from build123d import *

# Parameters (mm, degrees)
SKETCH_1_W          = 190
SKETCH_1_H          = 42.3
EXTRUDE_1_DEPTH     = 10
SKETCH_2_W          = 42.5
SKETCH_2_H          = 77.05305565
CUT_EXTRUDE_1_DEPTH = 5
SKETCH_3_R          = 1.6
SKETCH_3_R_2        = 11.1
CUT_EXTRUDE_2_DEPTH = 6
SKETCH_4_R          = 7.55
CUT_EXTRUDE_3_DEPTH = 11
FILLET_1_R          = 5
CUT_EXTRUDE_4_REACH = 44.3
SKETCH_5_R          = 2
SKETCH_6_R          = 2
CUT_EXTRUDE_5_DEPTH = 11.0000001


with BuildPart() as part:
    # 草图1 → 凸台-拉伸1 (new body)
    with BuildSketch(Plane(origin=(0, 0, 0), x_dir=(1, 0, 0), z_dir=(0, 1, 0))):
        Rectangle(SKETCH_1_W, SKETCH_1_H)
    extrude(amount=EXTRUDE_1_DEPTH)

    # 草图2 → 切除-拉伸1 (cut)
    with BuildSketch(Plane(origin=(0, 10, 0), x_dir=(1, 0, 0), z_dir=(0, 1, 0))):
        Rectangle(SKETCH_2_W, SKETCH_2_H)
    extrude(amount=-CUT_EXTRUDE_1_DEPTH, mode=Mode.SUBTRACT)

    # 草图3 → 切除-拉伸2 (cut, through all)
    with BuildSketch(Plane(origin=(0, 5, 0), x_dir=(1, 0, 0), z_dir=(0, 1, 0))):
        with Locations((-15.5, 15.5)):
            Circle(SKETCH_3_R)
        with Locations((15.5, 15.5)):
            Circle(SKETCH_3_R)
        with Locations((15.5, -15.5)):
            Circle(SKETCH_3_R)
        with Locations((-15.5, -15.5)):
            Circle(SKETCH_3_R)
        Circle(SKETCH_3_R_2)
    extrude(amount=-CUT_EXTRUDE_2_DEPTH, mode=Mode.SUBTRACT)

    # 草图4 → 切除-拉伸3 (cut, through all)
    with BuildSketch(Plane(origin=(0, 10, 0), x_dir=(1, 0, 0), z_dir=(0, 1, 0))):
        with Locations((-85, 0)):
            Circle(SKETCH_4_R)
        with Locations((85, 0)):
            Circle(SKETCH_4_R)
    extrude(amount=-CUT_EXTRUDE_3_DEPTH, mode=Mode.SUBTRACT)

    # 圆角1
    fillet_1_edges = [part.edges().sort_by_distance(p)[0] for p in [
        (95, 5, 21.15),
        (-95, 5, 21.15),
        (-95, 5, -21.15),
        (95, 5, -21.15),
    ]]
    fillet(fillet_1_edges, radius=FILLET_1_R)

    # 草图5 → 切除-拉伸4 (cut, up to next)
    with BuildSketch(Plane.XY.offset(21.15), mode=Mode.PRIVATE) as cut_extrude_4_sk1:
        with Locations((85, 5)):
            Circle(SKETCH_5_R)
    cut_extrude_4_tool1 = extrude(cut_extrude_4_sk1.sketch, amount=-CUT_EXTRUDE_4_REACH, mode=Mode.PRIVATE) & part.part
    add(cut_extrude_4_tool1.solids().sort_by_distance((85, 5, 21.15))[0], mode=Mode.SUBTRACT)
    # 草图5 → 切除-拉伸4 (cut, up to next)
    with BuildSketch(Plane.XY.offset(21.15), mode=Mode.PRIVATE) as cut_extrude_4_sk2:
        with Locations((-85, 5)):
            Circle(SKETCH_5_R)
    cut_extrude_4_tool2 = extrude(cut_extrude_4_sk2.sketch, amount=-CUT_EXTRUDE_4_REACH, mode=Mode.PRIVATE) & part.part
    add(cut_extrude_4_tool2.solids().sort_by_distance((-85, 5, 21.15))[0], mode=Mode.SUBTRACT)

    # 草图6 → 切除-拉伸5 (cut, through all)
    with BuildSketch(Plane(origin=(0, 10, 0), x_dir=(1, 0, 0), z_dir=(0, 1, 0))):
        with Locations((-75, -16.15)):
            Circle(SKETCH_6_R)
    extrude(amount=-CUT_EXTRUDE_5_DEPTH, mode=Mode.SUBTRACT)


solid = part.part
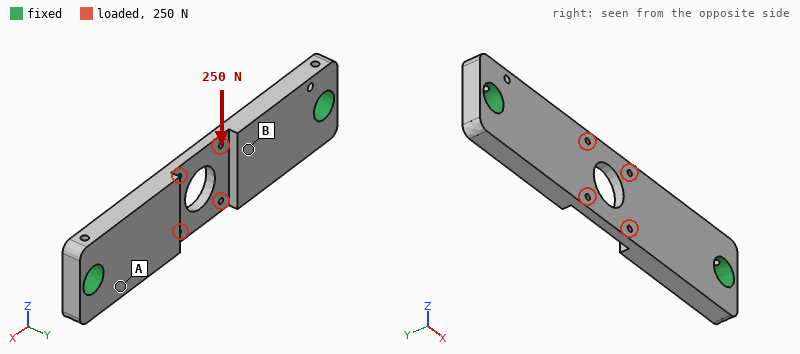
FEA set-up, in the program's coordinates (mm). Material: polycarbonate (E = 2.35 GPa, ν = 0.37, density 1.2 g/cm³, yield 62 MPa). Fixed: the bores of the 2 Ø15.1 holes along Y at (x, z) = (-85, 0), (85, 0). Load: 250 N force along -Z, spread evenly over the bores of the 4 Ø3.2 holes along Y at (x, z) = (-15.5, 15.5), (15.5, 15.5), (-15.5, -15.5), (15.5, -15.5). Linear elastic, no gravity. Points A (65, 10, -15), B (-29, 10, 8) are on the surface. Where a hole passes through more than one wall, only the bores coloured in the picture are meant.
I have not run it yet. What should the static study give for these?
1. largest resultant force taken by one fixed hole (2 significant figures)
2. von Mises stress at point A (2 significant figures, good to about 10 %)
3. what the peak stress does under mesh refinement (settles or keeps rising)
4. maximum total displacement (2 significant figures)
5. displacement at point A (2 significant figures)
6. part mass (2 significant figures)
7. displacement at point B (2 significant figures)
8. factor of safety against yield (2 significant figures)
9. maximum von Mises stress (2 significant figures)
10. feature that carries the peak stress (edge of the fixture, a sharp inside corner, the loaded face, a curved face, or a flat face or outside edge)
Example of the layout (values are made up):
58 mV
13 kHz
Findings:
130 N
0.76 MPa
settles
0.14 mm
0.031 mm
78 g
0.083 mm
11
5.8 MPa
the loaded face
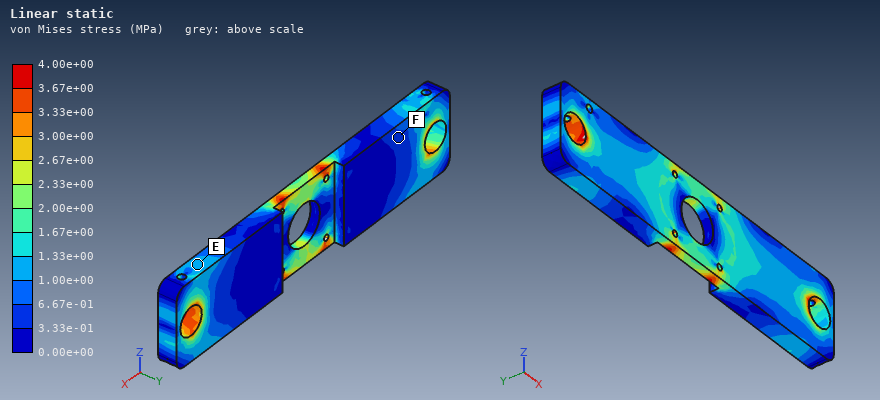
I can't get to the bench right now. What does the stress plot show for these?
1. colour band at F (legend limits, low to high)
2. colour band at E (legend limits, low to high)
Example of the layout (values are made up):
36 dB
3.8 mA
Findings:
3.33e-01 to 6.67e-01 MPa
1.00e+00 to 1.33e+00 MPa
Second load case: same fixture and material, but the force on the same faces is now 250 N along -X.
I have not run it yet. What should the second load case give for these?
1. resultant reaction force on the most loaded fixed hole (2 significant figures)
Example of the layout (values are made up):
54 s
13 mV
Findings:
130 N
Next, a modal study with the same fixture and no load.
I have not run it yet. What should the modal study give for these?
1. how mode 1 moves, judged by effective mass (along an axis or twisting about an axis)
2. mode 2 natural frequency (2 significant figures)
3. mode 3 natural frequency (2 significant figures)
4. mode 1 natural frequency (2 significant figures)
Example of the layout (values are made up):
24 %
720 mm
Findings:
along Y
1000 Hz
1300 Hz
540 Hz
